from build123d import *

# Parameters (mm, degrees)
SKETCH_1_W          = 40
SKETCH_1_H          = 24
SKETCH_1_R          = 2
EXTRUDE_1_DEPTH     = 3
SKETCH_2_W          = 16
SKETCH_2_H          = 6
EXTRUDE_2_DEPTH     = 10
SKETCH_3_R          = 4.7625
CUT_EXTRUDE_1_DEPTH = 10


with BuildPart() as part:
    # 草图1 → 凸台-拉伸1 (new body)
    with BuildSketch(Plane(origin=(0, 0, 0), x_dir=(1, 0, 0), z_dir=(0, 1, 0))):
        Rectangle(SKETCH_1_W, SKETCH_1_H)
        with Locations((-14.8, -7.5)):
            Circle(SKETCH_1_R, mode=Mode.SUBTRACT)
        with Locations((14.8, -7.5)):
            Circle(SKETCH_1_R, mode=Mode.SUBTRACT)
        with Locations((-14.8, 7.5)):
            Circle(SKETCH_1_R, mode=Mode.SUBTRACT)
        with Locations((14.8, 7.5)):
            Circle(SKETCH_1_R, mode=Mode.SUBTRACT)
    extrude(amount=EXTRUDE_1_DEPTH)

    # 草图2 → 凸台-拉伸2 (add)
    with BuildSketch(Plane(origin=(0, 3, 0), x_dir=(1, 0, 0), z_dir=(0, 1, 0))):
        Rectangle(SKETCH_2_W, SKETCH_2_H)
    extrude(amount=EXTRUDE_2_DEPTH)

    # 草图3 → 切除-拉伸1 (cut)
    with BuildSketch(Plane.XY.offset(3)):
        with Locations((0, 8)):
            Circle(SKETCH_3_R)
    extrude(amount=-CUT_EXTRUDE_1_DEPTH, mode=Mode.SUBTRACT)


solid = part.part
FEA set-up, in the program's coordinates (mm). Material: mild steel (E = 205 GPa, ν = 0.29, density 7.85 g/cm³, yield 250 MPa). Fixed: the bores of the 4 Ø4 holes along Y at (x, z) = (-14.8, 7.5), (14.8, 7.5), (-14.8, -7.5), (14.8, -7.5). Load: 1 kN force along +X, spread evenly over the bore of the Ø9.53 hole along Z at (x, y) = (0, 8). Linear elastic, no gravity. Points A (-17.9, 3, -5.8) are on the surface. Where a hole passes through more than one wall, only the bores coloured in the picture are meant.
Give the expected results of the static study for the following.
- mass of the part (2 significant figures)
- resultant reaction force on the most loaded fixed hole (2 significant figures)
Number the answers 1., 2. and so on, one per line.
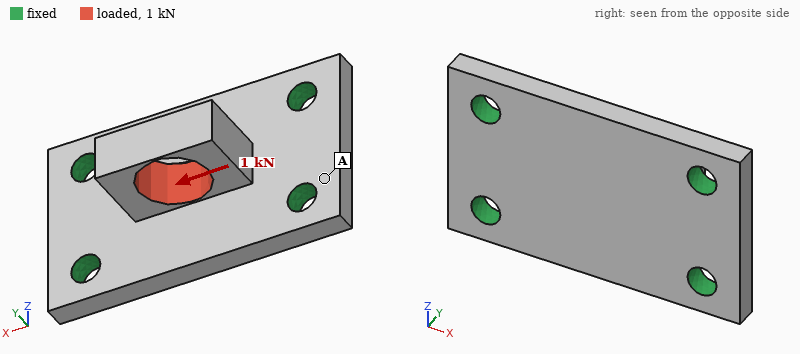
1. 26 g
2. 300 N
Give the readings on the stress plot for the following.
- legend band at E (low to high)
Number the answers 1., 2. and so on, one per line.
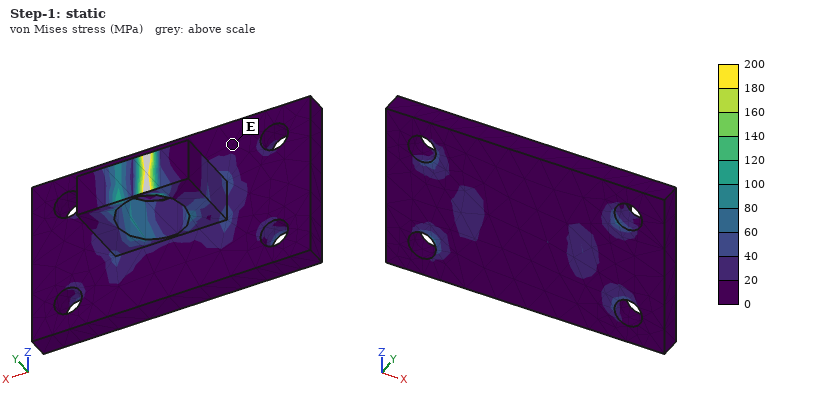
1. 0 to 20 MPa
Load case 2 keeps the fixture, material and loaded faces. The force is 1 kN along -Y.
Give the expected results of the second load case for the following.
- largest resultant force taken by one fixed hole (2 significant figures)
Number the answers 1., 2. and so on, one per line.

1. 260 N
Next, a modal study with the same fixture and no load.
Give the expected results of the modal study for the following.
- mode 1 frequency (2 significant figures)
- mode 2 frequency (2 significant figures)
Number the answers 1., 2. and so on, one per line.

1. 18 kHz
2. 19 kHz
